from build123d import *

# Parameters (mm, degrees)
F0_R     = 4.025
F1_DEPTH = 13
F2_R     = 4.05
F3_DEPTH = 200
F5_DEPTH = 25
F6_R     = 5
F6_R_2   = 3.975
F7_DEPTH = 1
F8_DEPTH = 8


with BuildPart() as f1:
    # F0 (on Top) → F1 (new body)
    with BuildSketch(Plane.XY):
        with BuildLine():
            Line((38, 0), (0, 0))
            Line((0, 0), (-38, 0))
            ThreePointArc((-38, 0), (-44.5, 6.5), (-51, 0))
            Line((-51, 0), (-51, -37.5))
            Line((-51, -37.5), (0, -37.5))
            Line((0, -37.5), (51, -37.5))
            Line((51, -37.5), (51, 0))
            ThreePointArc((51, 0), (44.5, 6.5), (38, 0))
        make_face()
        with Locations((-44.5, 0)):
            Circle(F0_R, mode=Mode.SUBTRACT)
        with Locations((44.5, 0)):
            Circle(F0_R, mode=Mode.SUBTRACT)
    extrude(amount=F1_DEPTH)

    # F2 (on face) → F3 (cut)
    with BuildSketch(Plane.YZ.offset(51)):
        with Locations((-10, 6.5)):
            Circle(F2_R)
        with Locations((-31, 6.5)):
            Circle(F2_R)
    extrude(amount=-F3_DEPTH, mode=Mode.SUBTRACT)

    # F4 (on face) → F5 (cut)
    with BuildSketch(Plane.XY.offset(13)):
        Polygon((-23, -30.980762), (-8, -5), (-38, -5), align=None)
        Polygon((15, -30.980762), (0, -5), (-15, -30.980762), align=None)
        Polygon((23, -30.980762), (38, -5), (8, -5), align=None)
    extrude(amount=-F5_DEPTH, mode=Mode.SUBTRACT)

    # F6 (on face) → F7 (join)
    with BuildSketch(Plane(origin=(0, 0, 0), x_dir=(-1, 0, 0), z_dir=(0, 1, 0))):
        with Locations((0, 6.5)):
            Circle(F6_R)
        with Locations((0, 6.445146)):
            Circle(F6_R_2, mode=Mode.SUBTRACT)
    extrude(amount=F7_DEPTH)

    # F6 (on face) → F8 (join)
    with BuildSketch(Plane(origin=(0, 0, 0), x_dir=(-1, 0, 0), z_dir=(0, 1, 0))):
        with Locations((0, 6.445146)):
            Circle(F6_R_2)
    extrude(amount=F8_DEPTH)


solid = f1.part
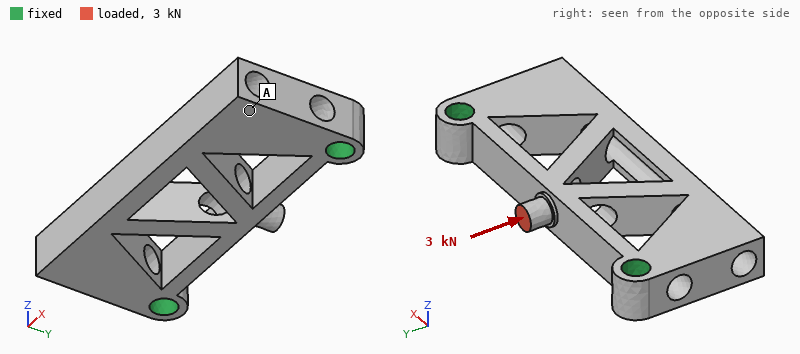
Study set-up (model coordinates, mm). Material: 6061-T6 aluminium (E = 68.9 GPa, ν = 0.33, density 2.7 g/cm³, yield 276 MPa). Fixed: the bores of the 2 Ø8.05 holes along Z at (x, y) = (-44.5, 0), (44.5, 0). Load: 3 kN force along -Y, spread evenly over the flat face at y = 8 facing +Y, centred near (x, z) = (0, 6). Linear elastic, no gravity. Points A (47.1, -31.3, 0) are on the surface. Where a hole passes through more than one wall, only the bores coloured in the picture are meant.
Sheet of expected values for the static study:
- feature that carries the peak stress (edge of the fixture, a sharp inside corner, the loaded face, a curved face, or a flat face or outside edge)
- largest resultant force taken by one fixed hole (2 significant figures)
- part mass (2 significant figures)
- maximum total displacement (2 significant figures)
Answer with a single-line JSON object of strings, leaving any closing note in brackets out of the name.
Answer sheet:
{"feature that carries the peak stress": "a curved face", "largest resultant force taken by one fixed hole": "1.8 kN", "part mass": "77 g", "maximum total displacement": "64 µm"}
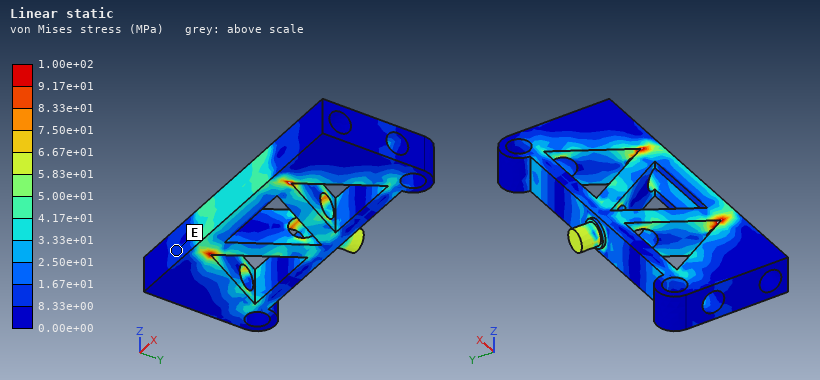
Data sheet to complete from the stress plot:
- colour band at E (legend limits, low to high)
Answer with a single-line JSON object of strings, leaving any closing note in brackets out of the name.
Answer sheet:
{"colour band at E": "8.33e+00 to 1.67e+01 MPa"}
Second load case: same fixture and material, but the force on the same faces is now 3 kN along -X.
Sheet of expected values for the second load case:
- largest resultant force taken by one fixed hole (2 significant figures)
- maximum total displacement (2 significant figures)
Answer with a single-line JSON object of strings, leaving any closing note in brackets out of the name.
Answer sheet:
{"largest resultant force taken by one fixed hole": "1.6 kN", "maximum total displacement": "0.15 mm"}
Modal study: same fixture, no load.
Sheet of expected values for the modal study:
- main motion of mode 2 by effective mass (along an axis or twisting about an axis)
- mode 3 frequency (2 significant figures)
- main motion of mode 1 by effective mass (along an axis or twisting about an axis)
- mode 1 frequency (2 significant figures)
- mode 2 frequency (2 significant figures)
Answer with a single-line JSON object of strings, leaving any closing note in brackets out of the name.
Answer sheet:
{"main motion of mode 2 by effective mass": "twisting about Y", "mode 3 frequency": "6900 Hz", "main motion of mode 1 by effective mass": "along Z", "mode 1 frequency": "4000 Hz", "mode 2 frequency": "6500 Hz"}
